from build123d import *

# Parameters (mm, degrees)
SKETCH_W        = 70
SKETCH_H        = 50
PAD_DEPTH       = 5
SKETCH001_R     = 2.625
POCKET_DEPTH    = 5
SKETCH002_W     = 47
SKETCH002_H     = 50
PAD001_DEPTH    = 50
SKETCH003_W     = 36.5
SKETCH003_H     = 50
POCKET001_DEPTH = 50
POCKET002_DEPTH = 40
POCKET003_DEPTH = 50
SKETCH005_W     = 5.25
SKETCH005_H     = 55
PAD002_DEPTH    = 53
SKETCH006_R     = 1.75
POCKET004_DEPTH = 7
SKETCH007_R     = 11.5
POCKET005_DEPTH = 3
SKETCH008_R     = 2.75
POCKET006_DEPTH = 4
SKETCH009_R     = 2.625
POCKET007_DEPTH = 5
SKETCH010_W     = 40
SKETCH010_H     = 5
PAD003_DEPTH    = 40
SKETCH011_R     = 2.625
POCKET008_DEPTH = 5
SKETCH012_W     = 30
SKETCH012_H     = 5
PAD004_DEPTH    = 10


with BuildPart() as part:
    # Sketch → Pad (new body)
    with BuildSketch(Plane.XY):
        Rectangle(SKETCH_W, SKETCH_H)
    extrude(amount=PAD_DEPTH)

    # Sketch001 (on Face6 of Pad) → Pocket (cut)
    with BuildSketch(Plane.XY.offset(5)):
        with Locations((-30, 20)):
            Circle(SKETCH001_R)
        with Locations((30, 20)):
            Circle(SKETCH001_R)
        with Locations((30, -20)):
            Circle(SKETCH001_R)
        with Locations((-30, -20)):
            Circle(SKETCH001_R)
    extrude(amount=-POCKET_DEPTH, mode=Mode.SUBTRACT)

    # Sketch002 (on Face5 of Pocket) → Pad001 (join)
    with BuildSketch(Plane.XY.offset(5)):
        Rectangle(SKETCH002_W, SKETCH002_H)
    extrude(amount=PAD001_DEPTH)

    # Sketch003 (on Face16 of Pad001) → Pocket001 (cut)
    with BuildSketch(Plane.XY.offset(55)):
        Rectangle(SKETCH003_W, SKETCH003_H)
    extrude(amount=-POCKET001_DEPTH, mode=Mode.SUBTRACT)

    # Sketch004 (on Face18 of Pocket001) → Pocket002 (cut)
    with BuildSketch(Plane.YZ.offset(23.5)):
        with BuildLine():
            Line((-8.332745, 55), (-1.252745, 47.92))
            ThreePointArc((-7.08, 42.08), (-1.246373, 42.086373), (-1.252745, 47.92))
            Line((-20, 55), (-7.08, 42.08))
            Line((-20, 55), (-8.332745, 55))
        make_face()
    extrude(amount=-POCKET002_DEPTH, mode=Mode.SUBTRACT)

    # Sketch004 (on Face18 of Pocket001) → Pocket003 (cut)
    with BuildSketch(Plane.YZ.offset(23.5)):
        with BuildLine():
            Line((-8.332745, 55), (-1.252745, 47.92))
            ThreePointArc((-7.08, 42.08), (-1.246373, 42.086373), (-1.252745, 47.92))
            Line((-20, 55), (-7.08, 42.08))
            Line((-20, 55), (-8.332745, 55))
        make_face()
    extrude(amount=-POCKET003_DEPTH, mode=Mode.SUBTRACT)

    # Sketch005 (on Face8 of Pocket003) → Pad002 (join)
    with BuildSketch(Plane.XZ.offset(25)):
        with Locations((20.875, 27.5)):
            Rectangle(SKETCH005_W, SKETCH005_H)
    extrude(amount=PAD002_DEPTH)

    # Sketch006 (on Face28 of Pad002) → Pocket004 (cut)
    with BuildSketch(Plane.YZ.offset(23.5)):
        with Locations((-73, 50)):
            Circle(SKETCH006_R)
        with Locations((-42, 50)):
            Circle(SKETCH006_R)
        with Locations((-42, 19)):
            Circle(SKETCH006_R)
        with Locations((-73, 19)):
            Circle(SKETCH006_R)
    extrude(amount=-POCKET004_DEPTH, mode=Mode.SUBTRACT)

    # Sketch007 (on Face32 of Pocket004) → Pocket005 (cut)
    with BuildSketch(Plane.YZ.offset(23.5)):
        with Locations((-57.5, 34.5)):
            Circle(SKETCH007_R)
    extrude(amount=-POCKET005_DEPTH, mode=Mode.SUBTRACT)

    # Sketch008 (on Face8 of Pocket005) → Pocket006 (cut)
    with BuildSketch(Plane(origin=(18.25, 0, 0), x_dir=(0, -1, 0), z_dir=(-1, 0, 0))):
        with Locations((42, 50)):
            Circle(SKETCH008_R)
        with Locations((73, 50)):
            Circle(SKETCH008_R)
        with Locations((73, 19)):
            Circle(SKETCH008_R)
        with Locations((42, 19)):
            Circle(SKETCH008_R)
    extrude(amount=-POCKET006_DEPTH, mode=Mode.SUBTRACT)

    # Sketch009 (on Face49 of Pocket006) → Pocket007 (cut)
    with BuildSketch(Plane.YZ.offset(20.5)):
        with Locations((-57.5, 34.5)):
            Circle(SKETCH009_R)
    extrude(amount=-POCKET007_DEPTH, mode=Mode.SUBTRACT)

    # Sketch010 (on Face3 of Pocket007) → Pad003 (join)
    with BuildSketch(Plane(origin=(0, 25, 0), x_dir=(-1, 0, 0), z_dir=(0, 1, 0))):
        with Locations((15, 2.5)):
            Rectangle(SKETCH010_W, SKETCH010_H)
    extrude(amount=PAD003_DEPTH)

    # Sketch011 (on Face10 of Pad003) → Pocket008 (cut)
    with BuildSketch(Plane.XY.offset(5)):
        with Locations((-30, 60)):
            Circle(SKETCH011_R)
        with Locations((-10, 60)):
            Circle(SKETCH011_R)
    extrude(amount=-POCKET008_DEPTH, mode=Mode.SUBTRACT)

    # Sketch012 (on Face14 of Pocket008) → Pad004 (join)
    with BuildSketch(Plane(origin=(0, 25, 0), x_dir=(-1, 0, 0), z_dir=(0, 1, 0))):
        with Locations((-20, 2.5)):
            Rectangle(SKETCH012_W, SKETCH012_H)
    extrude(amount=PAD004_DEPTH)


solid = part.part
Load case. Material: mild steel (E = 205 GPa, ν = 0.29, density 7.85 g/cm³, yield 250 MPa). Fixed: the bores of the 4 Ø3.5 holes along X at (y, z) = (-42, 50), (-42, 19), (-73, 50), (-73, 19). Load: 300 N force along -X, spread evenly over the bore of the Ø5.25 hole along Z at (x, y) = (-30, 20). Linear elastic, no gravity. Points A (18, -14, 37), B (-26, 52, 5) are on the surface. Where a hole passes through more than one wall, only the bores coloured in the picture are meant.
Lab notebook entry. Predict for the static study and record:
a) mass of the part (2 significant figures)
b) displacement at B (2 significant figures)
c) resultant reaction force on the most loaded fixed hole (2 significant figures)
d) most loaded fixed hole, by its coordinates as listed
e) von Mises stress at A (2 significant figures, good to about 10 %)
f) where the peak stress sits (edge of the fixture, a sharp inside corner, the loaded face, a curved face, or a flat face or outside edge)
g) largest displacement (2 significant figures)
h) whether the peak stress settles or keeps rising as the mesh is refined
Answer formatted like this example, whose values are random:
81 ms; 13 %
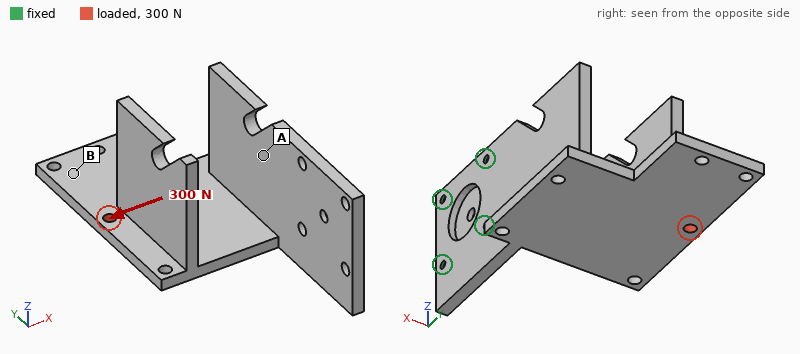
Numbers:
510 g; 0.48 mm; 1.5 kN; (-42, 19); 48 MPa; edge of the fixture; 0.56 mm; keeps rising
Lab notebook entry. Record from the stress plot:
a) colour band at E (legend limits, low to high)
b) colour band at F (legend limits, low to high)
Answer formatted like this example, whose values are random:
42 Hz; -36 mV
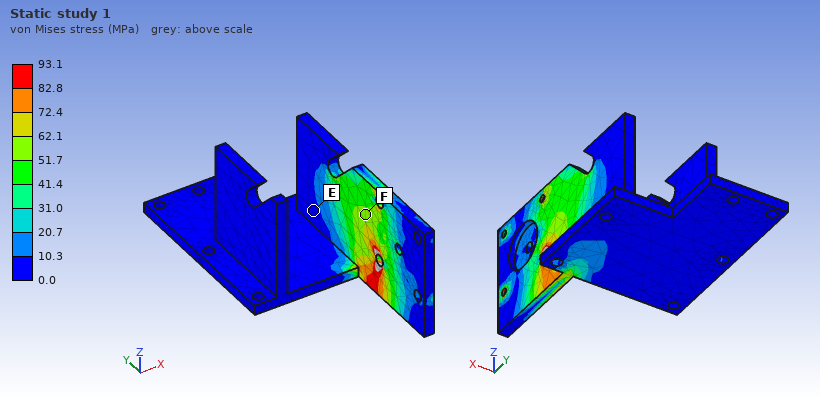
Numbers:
0.0 to 10.3 MPa; 51.7 to 62.1 MPa
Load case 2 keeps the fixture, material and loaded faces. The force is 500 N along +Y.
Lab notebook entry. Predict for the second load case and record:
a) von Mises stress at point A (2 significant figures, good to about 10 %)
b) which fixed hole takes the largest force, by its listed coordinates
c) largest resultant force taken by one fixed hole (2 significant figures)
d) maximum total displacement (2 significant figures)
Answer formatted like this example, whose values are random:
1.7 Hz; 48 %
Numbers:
73 MPa; (-73, 19); 1.6 kN; 0.87 mm
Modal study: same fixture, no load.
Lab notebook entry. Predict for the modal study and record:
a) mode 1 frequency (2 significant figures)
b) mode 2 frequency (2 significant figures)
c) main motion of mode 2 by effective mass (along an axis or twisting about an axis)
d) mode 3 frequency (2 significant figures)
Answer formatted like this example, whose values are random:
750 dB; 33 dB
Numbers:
260 Hz; 400 Hz; along Z; 990 Hz
